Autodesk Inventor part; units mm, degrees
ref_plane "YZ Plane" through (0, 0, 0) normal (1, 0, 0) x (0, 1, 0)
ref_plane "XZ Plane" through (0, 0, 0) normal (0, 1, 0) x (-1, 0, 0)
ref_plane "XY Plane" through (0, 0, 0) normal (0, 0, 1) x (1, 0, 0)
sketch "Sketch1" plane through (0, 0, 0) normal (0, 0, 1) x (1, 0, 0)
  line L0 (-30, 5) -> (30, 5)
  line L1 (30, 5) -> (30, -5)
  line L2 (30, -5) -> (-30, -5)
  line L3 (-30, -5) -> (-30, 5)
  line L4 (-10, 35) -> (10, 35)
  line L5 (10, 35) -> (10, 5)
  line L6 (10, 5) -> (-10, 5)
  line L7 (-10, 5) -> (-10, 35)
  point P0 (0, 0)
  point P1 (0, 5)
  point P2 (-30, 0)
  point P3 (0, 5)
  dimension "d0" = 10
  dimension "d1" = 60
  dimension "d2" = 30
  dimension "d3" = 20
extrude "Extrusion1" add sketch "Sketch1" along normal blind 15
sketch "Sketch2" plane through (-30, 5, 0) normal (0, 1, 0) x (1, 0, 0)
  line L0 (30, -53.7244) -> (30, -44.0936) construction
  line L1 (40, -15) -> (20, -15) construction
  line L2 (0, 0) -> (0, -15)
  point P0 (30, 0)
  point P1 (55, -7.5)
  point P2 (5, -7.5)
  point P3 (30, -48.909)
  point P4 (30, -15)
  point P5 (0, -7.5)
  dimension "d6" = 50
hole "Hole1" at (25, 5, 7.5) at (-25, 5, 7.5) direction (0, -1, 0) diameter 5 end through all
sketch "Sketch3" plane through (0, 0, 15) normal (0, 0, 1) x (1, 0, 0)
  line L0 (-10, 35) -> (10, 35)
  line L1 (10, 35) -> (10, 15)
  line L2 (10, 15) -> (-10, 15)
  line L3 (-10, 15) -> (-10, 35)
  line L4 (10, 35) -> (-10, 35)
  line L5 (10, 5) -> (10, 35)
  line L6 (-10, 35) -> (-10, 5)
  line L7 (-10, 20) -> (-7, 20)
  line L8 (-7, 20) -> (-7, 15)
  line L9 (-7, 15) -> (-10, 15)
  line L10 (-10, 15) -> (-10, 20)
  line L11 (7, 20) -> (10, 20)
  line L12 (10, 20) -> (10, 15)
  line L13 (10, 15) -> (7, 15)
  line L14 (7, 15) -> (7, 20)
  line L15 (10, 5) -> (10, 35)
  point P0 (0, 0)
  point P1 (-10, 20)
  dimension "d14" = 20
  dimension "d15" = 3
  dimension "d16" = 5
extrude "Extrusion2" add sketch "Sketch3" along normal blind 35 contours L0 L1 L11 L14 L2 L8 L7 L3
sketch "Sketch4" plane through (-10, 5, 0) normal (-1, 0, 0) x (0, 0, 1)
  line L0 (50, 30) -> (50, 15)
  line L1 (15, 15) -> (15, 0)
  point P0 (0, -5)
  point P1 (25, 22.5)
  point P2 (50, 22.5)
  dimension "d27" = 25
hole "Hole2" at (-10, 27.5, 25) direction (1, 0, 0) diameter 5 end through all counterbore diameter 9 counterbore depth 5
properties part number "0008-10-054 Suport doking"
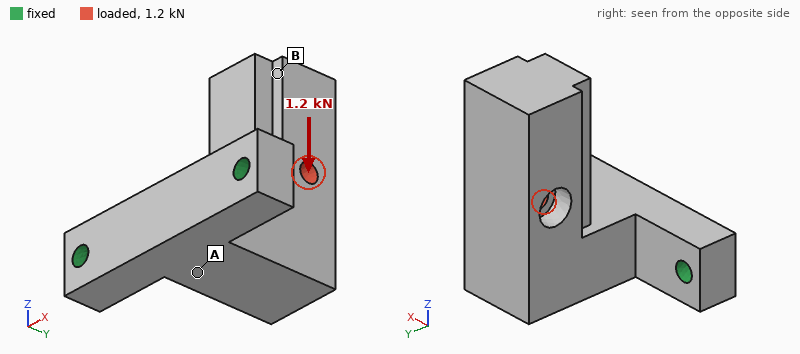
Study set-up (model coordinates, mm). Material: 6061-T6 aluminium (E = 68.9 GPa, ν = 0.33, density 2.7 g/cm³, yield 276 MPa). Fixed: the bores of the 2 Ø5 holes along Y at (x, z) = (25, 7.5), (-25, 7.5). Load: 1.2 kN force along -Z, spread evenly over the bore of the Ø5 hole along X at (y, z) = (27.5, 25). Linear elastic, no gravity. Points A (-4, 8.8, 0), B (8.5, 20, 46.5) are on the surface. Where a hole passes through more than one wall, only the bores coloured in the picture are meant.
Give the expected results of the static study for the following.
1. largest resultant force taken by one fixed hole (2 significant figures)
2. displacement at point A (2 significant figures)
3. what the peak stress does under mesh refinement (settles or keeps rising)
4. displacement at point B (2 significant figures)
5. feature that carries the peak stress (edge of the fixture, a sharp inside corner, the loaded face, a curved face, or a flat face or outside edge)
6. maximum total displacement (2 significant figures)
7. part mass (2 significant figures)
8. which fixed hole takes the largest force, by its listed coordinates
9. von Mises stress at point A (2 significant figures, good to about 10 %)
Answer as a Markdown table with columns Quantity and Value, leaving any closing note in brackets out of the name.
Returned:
| Quantity | Value |
|---|---|
| largest resultant force taken by one fixed hole | 670 N |
| displacement at point A | 0.051 mm |
| what the peak stress does under mesh refinement | keeps rising |
| displacement at point B | 0.20 mm |
| feature that carries the peak stress | edge of the fixture |
| maximum total displacement | 0.25 mm |
| part mass | 81 g |
| which fixed hole takes the largest force, by its listed coordinates | (25, 7.5) |
| von Mises stress at point A | 27 MPa |
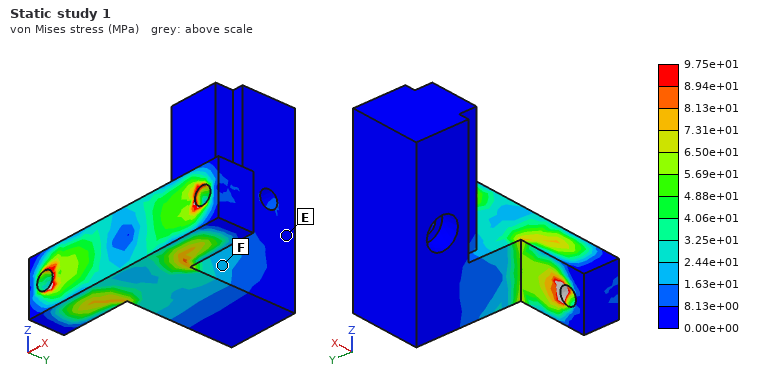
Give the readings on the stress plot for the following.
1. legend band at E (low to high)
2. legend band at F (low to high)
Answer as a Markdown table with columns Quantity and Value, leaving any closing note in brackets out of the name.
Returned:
| Quantity | Value |
|---|---|
| legend band at E | 0.00e+00 to 8.13e+00 MPa |
| legend band at F | 1.63e+01 to 2.44e+01 MPa |
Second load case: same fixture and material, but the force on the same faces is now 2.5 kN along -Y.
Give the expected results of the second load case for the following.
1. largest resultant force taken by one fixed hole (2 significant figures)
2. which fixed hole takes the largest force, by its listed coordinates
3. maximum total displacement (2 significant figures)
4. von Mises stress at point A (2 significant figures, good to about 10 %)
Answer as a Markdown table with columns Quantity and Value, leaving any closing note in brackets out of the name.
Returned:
| Quantity | Value |
|---|---|
| largest resultant force taken by one fixed hole | 1.5 kN |
| which fixed hole takes the largest force, by its listed coordinates | (25, 7.5) |
| maximum total displacement | 0.38 mm |
| von Mises stress at point A | 50 MPa |
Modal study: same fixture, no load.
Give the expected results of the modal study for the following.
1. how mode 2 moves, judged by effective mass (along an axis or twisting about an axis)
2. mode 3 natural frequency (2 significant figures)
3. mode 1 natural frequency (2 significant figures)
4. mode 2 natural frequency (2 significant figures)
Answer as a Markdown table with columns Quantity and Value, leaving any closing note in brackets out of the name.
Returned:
| Quantity | Value |
|---|---|
| how mode 2 moves, judged by effective mass | along X |
| mode 3 natural frequency | 6200 Hz |
| mode 1 natural frequency | 1700 Hz |
| mode 2 natural frequency | 3100 Hz |
